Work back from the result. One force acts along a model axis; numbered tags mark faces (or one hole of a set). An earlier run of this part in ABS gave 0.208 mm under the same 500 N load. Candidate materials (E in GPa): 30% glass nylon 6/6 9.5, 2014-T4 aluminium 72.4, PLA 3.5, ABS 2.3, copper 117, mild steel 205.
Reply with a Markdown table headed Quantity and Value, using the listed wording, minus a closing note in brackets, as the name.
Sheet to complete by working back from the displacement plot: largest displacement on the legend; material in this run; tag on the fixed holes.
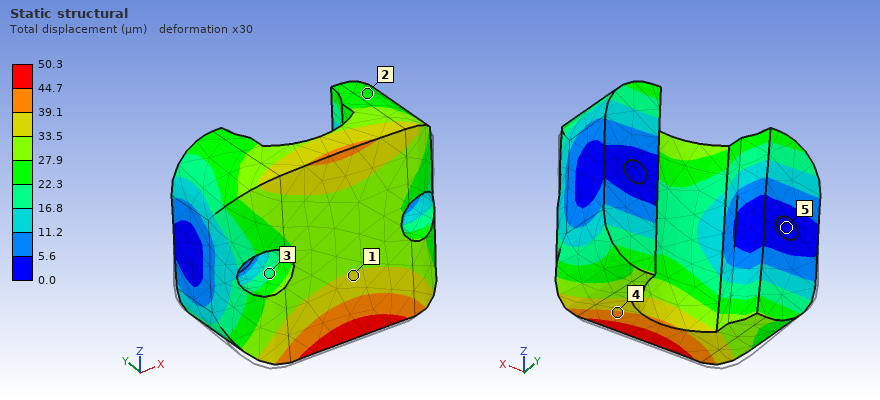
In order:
| Quantity | Value |
|---|---|
| largest displacement on the legend | 50.3 µm |
| material in this run | 30% glass nylon 6/6 |
| tag on the fixed holes | 5 |
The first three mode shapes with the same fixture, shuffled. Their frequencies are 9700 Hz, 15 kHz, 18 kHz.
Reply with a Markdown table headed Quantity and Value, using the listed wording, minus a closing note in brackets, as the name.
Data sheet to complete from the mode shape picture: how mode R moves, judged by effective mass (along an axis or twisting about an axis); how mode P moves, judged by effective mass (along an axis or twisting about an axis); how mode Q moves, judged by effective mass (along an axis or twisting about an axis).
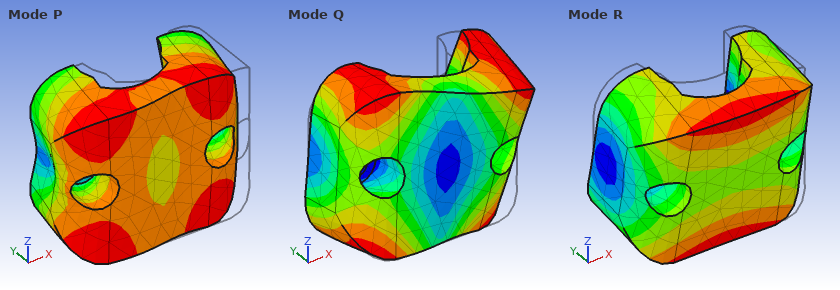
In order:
| Quantity | Value |
|---|---|
| how mode R moves, judged by effective mass | along Z |
| how mode P moves, judged by effective mass | along X |
| how mode Q moves, judged by effective mass | twisting about Y |
